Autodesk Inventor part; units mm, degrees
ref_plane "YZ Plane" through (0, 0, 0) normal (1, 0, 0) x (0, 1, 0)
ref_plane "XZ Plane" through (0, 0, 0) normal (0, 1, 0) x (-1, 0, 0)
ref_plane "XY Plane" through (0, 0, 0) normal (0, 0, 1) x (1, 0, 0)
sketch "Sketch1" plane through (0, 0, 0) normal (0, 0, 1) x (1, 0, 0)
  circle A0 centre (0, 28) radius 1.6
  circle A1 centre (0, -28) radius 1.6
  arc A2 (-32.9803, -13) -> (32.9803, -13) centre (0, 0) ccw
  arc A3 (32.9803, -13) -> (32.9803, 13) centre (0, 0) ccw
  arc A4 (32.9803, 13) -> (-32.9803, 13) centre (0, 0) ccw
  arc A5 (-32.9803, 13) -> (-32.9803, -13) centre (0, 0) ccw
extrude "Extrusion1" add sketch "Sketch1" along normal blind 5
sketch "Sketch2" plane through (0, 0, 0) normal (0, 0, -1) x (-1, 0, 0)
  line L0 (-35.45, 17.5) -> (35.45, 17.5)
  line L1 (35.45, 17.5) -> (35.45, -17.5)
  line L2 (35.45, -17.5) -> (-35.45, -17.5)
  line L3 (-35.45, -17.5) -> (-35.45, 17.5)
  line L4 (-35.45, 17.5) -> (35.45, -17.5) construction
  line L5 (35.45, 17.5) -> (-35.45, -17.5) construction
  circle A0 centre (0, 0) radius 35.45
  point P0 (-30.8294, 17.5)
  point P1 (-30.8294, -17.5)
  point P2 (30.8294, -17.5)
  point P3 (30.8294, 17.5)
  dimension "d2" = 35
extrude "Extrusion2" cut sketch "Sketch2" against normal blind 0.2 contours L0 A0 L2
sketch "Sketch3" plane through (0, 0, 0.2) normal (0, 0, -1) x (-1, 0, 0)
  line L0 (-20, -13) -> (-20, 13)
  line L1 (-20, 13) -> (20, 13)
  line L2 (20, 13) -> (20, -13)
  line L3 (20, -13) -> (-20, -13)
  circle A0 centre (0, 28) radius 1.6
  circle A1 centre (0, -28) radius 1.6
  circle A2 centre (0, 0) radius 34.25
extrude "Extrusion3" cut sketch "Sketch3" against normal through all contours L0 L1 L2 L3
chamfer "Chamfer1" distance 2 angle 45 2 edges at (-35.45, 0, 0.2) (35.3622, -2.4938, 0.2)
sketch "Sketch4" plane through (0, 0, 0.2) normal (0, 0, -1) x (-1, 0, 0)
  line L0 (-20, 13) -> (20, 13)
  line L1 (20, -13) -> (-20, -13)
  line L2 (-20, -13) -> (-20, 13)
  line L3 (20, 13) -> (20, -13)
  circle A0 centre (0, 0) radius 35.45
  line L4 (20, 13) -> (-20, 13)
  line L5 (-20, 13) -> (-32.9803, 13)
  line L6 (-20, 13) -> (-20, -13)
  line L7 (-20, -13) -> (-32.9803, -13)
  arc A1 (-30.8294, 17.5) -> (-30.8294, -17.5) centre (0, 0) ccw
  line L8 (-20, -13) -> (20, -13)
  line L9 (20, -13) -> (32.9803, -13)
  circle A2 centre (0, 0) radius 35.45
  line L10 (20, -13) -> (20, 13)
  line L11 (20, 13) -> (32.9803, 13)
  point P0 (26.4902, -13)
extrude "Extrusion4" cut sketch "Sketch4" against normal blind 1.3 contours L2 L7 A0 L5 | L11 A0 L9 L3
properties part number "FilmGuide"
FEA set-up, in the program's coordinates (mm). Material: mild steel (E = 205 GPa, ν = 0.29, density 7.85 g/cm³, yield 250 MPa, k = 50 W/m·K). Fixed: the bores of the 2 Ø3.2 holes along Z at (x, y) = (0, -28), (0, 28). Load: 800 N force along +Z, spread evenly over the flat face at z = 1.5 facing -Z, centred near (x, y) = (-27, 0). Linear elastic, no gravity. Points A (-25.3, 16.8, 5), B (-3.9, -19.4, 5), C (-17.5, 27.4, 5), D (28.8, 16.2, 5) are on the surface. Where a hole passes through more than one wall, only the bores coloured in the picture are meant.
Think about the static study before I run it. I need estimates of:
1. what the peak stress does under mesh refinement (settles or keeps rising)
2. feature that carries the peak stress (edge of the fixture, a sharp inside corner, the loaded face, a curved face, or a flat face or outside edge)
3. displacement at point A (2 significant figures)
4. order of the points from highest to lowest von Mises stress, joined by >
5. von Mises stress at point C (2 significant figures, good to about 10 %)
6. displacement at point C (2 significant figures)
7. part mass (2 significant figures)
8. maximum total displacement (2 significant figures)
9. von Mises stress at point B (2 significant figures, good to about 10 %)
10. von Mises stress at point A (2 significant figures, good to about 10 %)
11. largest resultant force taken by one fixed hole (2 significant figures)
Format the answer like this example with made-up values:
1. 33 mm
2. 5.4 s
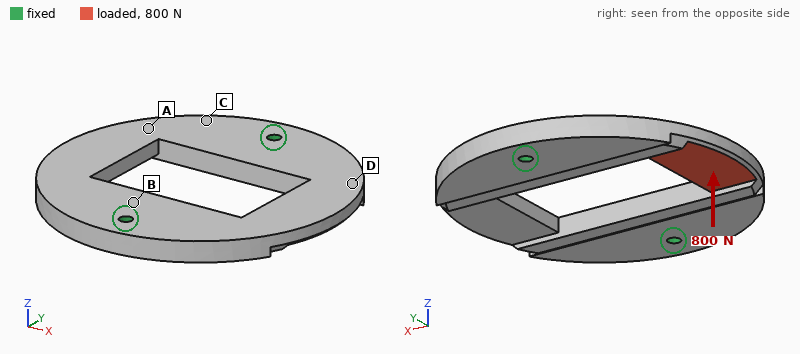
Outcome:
1. keeps rising
2. edge of the fixture
3. 0.089 mm
4. B > C > A > D
5. 71 MPa
6. 0.036 mm
7. 100 g
8. 0.17 mm
9. 93 MPa
10. 39 MPa
11. 430 N
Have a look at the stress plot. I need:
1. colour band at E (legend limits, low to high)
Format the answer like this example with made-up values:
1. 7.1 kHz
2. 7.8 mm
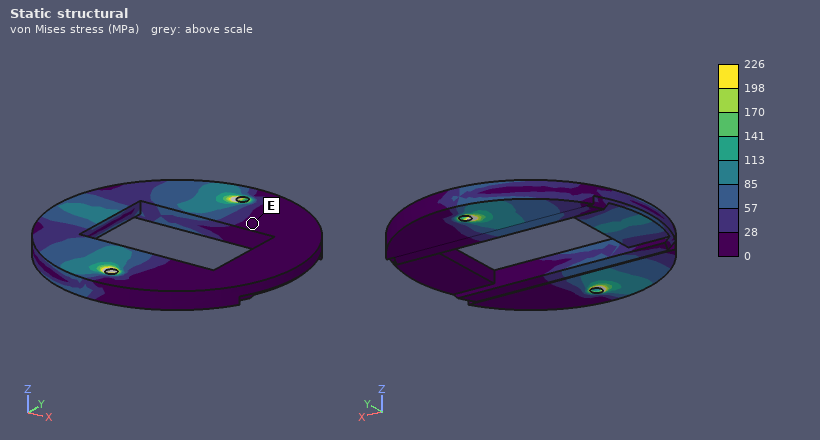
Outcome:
1. 0 to 28 MPa
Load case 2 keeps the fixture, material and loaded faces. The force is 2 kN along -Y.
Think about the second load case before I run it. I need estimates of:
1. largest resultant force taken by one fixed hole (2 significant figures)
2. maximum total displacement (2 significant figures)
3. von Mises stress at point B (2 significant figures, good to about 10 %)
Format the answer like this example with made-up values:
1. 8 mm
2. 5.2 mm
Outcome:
1. 1.3 kN
2. 19 µm
3. 15 MPa
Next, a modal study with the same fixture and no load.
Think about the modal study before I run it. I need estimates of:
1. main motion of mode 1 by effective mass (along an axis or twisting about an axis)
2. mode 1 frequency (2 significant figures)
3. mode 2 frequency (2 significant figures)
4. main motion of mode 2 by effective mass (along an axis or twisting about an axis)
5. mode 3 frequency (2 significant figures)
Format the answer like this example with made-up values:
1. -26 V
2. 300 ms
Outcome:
1. twisting about Y
2. 2800 Hz
3. 3500 Hz
4. along Z
5. 6100 Hz
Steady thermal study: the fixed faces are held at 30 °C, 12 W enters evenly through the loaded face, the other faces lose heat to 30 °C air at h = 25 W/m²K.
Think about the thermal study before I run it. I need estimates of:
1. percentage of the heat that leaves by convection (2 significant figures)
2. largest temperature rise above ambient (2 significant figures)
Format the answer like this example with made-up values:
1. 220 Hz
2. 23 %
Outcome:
1. 19 %
2. 58 K
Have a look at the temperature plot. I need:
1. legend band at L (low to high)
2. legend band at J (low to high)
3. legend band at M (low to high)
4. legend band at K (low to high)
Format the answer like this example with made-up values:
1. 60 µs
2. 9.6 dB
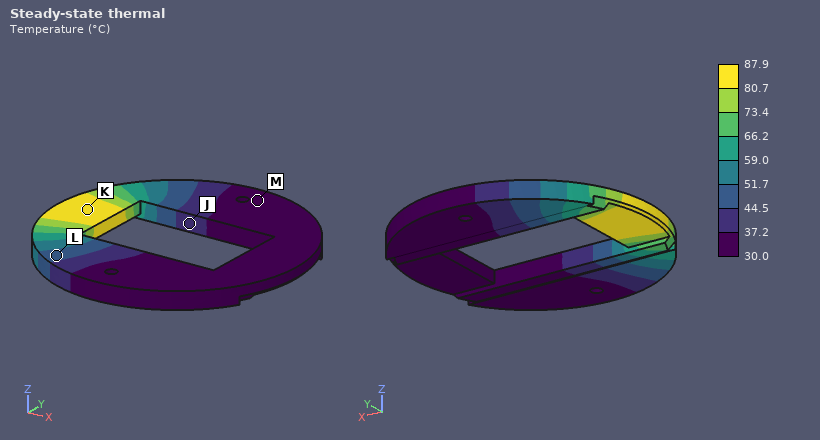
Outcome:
1. 44.5 to 51.7 °C
2. 37.2 to 44.5 °C
3. 30.0 to 37.2 °C
4. 80.7 to 87.9 °C
